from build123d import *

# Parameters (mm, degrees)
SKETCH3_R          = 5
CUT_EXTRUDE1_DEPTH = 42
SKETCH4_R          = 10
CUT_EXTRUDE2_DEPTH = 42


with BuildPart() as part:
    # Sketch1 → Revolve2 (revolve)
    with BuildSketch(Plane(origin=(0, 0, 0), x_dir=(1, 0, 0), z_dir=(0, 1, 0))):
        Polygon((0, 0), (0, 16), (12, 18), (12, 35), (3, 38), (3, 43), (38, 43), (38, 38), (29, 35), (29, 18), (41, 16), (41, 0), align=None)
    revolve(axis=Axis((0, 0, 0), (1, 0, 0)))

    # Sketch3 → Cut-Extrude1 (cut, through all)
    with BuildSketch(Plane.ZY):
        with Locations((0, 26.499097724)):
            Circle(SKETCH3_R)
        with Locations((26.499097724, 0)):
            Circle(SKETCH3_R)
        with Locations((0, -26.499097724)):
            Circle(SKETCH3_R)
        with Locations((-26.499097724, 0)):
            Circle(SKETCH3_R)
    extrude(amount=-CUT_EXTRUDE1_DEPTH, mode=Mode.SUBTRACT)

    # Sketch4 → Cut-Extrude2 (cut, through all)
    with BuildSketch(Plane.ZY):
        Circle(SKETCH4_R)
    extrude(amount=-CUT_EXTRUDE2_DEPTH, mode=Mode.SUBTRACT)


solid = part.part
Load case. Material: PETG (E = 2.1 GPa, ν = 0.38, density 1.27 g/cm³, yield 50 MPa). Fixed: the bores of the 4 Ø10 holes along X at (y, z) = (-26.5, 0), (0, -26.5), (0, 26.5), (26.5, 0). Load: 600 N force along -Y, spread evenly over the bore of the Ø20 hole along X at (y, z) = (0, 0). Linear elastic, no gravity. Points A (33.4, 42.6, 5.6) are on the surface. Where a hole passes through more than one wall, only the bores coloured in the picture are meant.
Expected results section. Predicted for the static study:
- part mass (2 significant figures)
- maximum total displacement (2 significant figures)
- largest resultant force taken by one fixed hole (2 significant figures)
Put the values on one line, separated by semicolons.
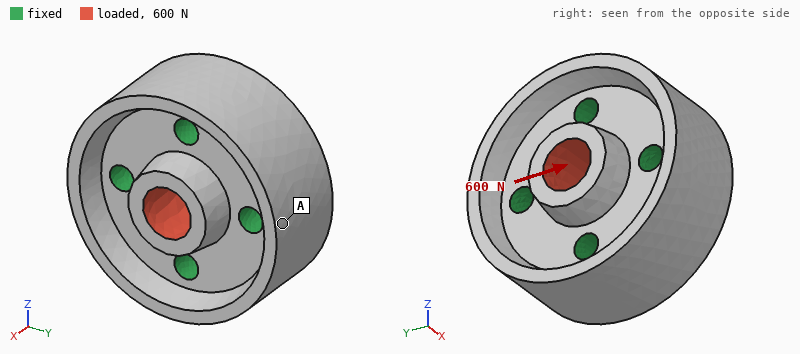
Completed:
170 g; 9.8 µm; 190 N
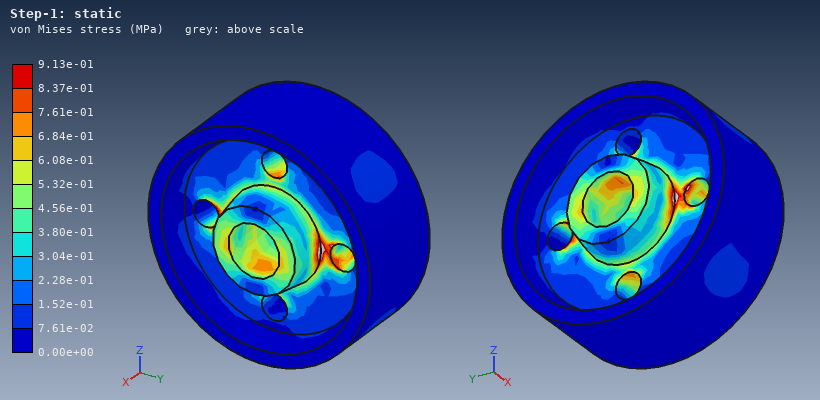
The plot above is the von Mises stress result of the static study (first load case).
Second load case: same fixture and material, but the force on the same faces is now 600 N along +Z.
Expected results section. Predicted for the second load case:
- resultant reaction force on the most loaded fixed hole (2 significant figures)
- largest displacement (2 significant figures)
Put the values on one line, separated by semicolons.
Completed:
190 N; 9.9 µm
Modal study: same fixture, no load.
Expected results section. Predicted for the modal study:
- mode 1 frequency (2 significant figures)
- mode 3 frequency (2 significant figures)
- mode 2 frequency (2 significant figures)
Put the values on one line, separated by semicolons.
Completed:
3900 Hz; 4300 Hz; 4300 Hz
